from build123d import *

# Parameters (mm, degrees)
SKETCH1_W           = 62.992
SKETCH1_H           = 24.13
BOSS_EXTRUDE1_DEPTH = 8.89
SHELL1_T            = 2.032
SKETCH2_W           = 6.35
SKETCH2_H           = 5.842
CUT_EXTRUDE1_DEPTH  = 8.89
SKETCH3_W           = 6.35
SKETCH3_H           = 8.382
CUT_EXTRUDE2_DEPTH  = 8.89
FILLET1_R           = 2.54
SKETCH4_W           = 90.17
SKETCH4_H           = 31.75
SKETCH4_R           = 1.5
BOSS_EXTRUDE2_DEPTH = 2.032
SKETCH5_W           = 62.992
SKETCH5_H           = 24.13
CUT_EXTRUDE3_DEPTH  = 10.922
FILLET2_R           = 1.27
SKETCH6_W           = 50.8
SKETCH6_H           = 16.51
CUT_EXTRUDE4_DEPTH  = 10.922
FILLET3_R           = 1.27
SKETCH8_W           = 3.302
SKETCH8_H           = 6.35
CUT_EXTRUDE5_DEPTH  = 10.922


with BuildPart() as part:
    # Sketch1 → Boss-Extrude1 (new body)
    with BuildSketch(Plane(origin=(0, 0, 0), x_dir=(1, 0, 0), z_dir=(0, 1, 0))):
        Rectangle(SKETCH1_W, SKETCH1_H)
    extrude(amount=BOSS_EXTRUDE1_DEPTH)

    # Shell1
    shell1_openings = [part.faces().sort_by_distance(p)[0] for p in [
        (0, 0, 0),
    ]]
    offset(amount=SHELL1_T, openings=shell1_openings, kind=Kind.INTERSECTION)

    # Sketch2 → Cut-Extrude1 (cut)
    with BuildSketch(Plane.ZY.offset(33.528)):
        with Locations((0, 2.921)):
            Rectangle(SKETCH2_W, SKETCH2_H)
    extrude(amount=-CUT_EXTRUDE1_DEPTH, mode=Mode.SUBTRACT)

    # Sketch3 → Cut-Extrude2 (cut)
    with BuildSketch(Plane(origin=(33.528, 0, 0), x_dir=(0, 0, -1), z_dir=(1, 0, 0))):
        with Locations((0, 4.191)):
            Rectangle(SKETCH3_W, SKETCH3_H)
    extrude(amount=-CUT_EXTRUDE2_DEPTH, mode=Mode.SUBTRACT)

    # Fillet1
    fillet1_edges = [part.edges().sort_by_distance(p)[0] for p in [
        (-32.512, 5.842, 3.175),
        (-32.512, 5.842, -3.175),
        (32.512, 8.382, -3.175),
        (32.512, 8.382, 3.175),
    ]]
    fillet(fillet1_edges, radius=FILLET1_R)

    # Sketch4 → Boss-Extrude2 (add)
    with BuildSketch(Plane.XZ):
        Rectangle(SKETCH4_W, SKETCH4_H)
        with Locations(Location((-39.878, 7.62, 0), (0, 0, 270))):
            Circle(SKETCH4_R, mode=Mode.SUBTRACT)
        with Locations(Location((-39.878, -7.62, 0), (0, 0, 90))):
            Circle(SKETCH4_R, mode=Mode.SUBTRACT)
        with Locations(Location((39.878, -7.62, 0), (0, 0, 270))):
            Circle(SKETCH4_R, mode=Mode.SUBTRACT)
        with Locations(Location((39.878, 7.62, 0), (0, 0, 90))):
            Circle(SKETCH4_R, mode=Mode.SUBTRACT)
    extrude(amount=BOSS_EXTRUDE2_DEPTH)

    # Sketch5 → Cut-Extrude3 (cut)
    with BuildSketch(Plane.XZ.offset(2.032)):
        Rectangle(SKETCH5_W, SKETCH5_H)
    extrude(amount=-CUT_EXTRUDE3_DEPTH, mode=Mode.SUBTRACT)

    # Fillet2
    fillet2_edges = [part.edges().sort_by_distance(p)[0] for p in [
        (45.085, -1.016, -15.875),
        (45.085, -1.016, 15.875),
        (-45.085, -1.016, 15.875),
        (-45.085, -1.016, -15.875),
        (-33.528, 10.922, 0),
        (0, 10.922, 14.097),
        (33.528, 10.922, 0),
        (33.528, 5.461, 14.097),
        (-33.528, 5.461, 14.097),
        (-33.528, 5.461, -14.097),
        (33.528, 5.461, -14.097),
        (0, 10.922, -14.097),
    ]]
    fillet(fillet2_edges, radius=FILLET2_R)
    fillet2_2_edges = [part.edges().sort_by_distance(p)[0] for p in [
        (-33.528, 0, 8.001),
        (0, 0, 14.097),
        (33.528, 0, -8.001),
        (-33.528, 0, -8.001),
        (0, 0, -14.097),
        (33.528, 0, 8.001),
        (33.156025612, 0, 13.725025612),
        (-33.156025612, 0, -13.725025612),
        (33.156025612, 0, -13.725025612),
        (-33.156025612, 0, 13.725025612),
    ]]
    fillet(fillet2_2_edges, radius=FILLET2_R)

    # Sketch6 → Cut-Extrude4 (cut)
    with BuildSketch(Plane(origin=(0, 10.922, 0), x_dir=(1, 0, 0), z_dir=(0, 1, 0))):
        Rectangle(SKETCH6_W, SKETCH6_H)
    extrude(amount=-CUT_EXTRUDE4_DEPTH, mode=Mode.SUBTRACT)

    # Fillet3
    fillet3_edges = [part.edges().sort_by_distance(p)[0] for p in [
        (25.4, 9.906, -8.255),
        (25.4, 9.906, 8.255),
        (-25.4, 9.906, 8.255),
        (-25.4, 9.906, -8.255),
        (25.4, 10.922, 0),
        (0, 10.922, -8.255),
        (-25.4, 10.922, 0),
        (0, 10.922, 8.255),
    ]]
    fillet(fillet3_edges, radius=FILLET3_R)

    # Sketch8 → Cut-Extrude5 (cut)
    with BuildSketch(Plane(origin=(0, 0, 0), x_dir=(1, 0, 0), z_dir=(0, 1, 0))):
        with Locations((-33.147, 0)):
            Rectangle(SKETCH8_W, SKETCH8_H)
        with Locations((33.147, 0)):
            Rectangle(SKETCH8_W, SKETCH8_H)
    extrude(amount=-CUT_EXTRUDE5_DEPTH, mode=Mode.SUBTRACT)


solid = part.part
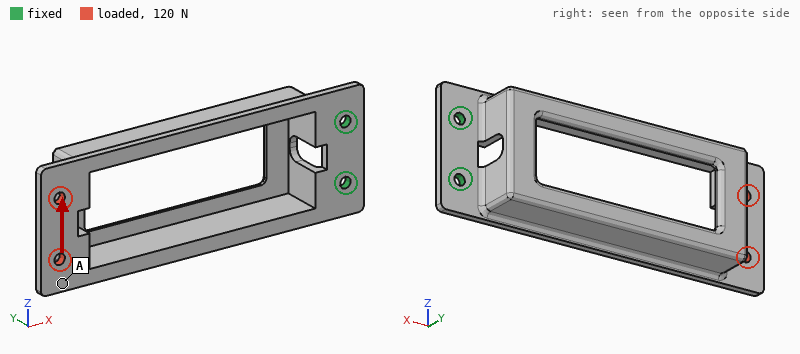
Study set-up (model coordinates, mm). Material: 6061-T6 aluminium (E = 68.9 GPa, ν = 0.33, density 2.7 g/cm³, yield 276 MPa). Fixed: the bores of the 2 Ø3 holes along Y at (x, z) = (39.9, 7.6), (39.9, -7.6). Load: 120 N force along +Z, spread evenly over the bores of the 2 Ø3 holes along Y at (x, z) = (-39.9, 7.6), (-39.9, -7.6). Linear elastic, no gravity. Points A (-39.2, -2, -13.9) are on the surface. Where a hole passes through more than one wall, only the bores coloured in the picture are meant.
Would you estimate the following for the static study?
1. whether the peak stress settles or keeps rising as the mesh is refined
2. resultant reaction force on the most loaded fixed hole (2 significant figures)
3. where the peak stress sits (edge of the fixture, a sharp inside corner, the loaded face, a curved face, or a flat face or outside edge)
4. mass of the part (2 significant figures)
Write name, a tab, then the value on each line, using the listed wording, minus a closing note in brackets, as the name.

whether the peak stress settles or keeps rising as the mesh is refined	keeps rising
resultant reaction force on the most loaded fixed hole	490 N
where the peak stress sits	edge of the fixture
mass of the part	21 g
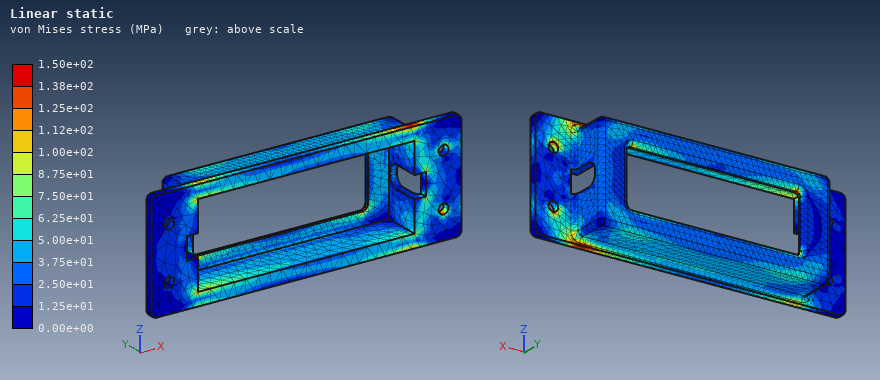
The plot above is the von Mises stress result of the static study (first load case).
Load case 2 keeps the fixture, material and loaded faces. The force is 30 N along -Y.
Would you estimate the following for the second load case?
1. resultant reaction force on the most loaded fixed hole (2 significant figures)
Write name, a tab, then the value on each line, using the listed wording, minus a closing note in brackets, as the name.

resultant reaction force on the most loaded fixed hole	36 N
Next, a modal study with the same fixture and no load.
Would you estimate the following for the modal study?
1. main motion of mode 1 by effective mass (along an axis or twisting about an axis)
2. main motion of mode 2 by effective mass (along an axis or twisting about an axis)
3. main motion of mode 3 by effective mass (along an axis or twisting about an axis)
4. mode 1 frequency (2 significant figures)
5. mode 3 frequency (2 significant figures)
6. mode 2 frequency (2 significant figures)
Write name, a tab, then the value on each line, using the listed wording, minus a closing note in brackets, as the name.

main motion of mode 1 by effective mass	along Y
main motion of mode 2 by effective mass	along Z
main motion of mode 3 by effective mass	along Z
mode 1 frequency	320 Hz
mode 3 frequency	1900 Hz
mode 2 frequency	730 Hz
